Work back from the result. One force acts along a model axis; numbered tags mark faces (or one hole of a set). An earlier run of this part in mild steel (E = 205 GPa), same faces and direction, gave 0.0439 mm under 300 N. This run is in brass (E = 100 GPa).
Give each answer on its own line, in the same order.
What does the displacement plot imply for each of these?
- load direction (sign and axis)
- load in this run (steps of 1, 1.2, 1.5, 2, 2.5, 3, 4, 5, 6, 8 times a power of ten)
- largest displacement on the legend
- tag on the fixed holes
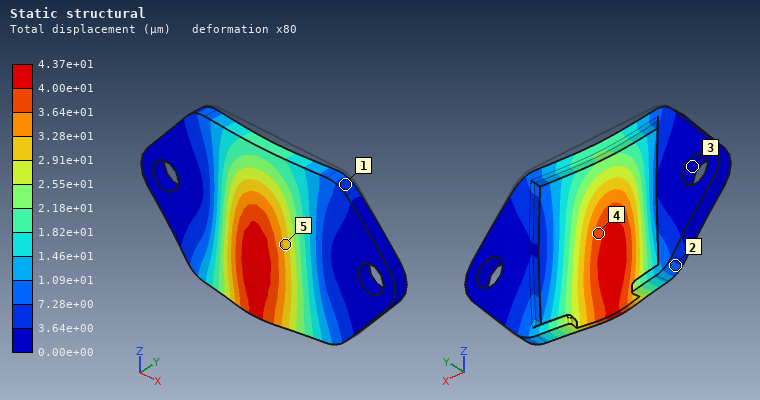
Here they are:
-Y
150 N
4.37e+01 µm
3
